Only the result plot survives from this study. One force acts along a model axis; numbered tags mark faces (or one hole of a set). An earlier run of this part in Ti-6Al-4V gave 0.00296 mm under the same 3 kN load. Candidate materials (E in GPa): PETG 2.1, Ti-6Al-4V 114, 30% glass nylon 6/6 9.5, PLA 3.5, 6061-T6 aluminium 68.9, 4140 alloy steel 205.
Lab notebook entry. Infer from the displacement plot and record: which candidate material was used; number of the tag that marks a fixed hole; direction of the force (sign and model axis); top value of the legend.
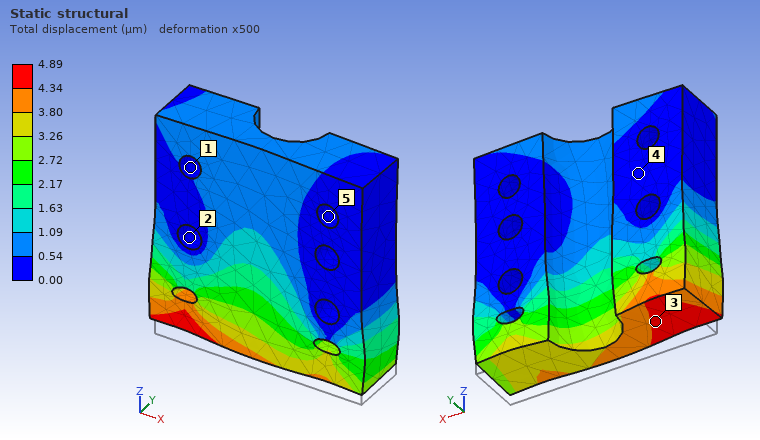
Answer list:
6061-T6 aluminium
2
+Z
4.89 µm
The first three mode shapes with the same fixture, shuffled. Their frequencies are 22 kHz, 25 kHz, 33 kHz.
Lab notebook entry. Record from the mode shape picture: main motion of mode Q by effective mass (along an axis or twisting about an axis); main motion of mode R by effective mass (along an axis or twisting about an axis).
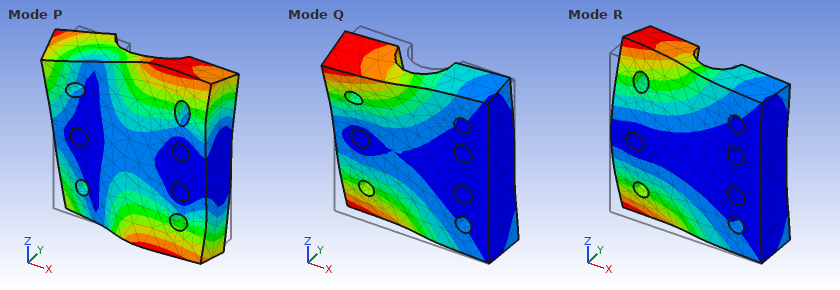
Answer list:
twisting about X
along Y
